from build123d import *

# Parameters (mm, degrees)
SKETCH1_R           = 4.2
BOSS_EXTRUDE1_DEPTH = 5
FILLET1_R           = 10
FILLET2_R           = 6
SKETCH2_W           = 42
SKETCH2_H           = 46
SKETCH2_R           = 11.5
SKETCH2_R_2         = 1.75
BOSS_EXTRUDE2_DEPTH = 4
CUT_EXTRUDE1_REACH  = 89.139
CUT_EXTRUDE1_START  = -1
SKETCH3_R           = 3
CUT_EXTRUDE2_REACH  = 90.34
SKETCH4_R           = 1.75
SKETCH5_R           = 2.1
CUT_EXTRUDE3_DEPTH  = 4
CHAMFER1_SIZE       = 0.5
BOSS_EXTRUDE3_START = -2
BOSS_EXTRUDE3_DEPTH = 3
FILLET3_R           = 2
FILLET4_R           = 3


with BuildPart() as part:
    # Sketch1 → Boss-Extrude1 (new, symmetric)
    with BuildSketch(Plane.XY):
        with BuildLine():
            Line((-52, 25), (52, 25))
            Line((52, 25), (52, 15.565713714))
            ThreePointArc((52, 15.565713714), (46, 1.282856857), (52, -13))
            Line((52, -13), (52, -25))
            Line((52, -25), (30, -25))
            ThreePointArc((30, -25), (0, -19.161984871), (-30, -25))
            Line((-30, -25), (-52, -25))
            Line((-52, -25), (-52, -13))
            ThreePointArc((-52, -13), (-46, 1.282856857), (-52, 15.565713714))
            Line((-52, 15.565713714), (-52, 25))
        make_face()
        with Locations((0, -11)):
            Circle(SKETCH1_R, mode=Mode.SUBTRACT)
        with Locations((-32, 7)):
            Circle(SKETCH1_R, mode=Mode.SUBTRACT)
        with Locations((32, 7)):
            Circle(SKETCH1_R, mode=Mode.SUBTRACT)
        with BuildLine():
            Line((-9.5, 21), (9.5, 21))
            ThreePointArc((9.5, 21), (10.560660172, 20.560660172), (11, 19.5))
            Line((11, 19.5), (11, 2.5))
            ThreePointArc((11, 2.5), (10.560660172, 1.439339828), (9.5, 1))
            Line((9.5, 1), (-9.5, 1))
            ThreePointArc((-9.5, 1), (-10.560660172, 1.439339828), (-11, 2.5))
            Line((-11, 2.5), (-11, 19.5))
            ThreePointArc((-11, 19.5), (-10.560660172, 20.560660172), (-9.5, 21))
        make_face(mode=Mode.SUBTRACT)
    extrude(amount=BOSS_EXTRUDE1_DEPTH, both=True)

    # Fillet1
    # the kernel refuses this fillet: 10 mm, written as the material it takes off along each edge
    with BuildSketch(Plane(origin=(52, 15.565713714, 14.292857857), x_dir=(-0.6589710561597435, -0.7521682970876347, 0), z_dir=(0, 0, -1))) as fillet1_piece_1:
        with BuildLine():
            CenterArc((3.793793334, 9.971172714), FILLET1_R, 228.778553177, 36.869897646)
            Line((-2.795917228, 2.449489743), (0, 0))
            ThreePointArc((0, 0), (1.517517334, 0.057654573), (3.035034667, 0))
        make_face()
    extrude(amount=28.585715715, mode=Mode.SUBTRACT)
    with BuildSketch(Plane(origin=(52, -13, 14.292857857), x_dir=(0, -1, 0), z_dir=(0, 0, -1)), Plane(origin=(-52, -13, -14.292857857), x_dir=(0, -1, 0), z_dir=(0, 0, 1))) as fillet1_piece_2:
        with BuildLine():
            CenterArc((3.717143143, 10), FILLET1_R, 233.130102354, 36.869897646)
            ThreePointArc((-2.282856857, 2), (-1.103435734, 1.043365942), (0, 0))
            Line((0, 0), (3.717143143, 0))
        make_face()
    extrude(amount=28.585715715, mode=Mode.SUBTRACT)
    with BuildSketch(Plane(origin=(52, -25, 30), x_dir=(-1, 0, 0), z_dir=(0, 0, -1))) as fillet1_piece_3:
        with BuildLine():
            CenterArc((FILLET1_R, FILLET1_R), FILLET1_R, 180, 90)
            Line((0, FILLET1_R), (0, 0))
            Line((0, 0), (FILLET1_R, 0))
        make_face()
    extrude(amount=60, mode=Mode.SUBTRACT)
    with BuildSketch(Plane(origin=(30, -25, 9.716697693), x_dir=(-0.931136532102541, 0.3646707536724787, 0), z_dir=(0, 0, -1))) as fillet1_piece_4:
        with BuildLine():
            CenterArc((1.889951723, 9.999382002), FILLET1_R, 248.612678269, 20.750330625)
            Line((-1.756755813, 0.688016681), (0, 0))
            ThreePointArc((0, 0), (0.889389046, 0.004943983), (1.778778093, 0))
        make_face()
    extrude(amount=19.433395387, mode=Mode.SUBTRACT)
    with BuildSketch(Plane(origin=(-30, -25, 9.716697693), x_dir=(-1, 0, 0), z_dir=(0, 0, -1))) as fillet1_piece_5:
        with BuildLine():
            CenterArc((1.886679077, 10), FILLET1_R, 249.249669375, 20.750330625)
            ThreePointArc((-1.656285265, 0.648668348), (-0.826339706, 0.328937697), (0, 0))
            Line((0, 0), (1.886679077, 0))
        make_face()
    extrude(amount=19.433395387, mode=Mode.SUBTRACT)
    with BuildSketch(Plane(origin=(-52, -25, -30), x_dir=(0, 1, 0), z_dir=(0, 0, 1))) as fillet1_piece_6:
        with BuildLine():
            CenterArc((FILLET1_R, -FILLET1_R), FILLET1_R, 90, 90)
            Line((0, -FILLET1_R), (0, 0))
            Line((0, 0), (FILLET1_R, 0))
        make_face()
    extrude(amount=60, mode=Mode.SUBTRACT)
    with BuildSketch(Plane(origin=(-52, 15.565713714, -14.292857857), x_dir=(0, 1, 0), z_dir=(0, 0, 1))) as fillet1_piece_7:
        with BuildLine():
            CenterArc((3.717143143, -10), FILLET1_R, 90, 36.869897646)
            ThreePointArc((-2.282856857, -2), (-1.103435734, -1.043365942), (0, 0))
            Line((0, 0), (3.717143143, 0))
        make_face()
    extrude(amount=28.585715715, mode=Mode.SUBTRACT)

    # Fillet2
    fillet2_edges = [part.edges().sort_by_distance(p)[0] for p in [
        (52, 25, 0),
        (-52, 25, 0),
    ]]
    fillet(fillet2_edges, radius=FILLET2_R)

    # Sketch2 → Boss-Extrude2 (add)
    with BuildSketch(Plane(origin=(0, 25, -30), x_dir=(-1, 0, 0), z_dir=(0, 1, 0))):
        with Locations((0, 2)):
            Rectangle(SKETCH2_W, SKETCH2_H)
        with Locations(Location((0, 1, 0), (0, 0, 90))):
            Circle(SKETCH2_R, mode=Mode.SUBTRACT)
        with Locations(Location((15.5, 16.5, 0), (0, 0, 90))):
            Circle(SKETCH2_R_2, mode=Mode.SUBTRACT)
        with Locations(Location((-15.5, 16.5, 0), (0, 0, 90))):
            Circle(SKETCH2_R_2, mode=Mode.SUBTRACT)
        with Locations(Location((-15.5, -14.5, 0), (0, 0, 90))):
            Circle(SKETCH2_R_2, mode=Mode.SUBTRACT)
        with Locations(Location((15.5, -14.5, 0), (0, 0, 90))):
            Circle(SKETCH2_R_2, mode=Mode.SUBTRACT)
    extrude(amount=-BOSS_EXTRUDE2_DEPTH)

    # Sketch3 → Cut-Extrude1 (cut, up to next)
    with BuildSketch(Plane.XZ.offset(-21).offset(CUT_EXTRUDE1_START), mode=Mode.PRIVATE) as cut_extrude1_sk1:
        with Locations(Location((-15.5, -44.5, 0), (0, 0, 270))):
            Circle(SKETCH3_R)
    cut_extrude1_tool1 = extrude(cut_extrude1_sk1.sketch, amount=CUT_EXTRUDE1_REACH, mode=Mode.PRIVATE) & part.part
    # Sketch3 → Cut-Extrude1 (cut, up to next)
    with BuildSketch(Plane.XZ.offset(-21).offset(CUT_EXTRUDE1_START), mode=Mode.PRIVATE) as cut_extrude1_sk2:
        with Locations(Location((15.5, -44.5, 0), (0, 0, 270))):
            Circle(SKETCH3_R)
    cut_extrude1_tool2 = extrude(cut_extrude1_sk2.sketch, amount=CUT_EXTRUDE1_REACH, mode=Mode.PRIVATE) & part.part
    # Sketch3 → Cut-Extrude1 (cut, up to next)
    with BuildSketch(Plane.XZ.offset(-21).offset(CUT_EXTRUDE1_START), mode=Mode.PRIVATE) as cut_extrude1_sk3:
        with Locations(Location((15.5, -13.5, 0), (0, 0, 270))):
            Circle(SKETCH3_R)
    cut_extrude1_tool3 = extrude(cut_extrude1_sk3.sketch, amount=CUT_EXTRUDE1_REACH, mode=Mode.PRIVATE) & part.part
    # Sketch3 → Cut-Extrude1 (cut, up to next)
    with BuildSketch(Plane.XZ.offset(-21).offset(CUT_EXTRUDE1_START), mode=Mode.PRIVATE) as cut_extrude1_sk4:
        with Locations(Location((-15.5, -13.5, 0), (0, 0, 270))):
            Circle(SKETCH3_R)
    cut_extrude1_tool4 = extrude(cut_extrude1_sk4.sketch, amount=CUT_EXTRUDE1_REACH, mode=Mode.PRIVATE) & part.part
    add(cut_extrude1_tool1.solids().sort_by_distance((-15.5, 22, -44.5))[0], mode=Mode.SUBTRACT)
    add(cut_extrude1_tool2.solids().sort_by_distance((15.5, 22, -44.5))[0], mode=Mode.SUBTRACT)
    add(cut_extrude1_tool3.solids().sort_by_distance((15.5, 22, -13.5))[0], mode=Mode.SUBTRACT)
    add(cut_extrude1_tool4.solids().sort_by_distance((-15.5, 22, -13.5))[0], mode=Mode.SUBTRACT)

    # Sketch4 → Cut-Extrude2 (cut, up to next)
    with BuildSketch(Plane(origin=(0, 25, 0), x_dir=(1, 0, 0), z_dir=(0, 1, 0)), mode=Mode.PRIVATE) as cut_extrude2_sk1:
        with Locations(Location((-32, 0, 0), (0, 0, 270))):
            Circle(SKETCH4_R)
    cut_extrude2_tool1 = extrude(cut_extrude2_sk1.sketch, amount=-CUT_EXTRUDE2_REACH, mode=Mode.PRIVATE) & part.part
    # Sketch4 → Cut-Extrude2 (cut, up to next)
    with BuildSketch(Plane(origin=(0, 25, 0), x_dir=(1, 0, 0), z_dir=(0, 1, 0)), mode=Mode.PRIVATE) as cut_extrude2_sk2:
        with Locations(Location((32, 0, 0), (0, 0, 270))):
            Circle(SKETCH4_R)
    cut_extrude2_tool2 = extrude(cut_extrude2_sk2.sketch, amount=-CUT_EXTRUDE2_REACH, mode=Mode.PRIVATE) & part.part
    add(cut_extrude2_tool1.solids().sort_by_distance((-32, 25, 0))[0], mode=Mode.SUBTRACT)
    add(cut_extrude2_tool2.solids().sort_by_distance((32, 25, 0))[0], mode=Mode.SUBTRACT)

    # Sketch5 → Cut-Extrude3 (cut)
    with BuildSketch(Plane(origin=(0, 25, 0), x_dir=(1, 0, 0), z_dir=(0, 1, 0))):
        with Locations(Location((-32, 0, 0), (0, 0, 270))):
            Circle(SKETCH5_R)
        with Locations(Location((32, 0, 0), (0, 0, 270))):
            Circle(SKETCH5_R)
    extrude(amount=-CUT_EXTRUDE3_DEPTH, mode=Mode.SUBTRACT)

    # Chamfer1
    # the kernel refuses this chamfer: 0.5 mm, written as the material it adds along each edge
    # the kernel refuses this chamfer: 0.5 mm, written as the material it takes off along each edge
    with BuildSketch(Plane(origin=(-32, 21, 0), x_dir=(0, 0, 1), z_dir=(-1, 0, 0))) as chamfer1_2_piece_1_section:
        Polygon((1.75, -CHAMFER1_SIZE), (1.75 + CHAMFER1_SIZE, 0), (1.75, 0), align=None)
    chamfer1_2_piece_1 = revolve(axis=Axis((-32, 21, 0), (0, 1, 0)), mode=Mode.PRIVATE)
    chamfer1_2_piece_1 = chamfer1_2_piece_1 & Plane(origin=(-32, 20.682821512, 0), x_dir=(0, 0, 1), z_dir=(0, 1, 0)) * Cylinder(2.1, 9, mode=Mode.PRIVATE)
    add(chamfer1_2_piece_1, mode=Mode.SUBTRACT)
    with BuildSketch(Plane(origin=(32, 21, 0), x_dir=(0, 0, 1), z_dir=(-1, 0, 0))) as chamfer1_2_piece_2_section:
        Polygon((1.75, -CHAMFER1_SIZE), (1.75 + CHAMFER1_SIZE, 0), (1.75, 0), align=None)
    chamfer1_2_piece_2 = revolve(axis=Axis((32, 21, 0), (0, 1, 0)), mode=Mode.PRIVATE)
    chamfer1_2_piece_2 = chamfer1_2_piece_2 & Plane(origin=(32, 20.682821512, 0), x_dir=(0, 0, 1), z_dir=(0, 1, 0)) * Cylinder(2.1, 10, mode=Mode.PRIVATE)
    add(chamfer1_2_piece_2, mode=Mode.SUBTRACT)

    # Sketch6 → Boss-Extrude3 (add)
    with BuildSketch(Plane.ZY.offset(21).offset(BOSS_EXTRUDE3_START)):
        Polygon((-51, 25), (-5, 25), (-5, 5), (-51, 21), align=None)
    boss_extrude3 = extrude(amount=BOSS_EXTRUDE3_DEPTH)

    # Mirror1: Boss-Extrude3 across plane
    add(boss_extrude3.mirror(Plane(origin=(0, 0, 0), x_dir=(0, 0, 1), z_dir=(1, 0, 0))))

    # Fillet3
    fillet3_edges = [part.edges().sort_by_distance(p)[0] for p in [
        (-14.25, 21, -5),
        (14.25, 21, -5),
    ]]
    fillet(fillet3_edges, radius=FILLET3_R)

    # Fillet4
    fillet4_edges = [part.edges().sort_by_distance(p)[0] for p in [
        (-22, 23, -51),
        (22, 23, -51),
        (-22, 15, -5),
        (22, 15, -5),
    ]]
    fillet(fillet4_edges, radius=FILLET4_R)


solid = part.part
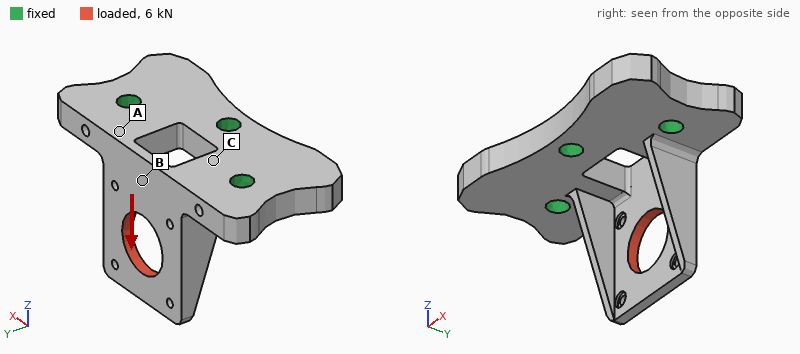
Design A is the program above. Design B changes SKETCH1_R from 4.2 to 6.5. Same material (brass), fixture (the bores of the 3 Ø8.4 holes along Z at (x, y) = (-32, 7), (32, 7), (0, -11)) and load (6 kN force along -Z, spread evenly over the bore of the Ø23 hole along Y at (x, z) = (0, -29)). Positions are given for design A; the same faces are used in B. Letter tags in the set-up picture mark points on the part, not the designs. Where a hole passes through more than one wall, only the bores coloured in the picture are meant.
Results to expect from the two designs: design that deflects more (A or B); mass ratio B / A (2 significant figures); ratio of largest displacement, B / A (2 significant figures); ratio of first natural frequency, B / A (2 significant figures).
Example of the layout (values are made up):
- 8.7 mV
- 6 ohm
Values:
- A
- 0.95
- 0.82
- 1.0
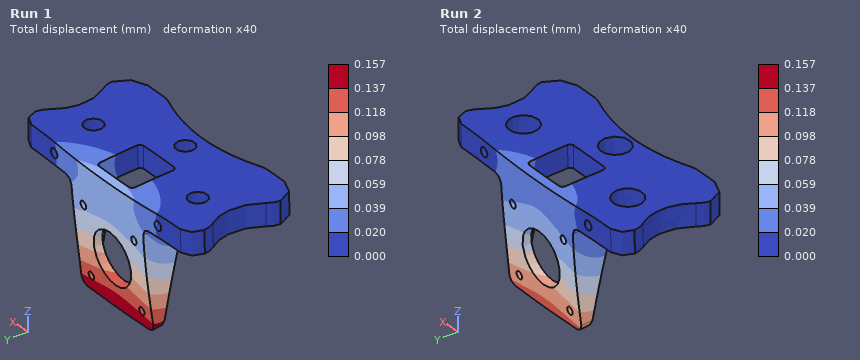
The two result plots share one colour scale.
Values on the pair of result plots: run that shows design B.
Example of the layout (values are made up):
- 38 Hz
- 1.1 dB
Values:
- Run 2
